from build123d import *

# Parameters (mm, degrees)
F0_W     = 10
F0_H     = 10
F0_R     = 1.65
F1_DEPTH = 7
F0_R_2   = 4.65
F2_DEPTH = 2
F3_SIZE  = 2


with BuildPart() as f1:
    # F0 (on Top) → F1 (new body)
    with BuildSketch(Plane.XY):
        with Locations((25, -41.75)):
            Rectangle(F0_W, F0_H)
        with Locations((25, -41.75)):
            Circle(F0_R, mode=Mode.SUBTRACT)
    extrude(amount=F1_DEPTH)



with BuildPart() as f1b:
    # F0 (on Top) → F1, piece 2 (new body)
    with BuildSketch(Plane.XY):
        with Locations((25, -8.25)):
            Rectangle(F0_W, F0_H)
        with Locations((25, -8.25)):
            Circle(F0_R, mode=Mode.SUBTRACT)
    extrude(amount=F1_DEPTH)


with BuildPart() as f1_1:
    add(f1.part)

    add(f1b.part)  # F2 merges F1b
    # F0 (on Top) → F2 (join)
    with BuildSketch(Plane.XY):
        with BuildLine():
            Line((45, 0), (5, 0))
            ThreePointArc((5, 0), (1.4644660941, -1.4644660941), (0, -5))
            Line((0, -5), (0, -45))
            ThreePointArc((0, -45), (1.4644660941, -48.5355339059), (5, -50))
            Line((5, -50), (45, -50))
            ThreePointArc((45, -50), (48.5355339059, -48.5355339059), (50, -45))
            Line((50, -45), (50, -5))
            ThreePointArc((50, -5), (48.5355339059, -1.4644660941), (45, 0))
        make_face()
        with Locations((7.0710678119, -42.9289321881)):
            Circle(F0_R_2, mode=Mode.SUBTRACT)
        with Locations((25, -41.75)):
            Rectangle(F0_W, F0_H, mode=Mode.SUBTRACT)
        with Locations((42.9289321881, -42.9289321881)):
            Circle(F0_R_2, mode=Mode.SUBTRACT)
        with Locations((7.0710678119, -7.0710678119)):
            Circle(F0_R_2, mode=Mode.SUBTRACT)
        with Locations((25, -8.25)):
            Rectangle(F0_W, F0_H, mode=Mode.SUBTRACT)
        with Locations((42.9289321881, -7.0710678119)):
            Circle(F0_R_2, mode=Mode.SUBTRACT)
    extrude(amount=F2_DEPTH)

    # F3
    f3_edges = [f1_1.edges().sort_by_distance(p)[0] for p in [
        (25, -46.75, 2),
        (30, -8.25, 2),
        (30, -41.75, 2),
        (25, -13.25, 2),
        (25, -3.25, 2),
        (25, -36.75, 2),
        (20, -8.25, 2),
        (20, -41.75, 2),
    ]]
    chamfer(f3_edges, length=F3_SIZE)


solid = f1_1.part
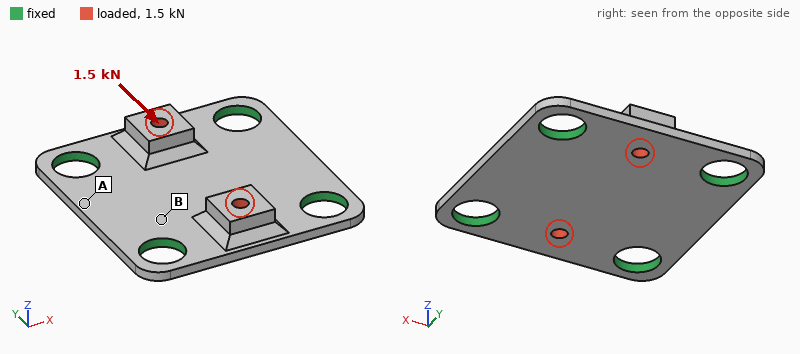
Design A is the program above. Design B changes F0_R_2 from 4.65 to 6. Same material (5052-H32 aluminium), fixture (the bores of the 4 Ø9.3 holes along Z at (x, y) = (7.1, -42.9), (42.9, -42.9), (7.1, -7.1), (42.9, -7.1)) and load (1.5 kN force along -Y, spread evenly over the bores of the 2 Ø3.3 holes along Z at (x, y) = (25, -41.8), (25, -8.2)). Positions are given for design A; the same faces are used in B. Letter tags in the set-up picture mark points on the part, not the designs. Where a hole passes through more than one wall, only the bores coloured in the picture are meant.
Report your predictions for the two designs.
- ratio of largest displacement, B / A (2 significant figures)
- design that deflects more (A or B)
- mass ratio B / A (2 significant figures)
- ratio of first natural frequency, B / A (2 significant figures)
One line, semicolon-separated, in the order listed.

0.80; A; 0.93; 1.2
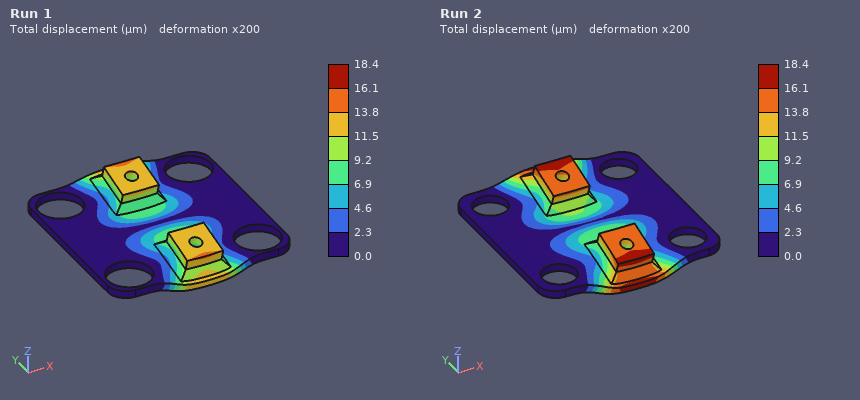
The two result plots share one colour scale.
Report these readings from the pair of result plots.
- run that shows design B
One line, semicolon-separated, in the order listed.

Run 1
